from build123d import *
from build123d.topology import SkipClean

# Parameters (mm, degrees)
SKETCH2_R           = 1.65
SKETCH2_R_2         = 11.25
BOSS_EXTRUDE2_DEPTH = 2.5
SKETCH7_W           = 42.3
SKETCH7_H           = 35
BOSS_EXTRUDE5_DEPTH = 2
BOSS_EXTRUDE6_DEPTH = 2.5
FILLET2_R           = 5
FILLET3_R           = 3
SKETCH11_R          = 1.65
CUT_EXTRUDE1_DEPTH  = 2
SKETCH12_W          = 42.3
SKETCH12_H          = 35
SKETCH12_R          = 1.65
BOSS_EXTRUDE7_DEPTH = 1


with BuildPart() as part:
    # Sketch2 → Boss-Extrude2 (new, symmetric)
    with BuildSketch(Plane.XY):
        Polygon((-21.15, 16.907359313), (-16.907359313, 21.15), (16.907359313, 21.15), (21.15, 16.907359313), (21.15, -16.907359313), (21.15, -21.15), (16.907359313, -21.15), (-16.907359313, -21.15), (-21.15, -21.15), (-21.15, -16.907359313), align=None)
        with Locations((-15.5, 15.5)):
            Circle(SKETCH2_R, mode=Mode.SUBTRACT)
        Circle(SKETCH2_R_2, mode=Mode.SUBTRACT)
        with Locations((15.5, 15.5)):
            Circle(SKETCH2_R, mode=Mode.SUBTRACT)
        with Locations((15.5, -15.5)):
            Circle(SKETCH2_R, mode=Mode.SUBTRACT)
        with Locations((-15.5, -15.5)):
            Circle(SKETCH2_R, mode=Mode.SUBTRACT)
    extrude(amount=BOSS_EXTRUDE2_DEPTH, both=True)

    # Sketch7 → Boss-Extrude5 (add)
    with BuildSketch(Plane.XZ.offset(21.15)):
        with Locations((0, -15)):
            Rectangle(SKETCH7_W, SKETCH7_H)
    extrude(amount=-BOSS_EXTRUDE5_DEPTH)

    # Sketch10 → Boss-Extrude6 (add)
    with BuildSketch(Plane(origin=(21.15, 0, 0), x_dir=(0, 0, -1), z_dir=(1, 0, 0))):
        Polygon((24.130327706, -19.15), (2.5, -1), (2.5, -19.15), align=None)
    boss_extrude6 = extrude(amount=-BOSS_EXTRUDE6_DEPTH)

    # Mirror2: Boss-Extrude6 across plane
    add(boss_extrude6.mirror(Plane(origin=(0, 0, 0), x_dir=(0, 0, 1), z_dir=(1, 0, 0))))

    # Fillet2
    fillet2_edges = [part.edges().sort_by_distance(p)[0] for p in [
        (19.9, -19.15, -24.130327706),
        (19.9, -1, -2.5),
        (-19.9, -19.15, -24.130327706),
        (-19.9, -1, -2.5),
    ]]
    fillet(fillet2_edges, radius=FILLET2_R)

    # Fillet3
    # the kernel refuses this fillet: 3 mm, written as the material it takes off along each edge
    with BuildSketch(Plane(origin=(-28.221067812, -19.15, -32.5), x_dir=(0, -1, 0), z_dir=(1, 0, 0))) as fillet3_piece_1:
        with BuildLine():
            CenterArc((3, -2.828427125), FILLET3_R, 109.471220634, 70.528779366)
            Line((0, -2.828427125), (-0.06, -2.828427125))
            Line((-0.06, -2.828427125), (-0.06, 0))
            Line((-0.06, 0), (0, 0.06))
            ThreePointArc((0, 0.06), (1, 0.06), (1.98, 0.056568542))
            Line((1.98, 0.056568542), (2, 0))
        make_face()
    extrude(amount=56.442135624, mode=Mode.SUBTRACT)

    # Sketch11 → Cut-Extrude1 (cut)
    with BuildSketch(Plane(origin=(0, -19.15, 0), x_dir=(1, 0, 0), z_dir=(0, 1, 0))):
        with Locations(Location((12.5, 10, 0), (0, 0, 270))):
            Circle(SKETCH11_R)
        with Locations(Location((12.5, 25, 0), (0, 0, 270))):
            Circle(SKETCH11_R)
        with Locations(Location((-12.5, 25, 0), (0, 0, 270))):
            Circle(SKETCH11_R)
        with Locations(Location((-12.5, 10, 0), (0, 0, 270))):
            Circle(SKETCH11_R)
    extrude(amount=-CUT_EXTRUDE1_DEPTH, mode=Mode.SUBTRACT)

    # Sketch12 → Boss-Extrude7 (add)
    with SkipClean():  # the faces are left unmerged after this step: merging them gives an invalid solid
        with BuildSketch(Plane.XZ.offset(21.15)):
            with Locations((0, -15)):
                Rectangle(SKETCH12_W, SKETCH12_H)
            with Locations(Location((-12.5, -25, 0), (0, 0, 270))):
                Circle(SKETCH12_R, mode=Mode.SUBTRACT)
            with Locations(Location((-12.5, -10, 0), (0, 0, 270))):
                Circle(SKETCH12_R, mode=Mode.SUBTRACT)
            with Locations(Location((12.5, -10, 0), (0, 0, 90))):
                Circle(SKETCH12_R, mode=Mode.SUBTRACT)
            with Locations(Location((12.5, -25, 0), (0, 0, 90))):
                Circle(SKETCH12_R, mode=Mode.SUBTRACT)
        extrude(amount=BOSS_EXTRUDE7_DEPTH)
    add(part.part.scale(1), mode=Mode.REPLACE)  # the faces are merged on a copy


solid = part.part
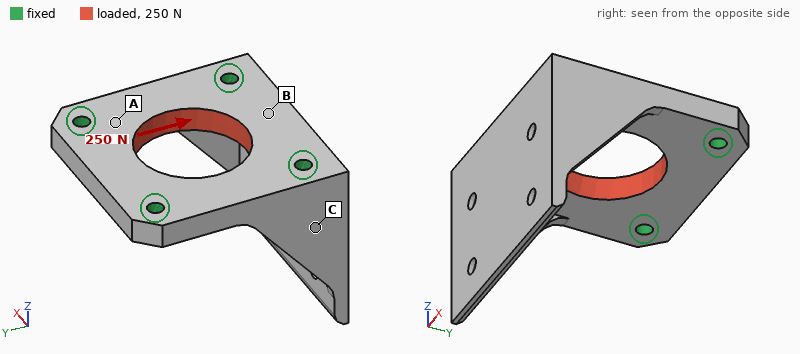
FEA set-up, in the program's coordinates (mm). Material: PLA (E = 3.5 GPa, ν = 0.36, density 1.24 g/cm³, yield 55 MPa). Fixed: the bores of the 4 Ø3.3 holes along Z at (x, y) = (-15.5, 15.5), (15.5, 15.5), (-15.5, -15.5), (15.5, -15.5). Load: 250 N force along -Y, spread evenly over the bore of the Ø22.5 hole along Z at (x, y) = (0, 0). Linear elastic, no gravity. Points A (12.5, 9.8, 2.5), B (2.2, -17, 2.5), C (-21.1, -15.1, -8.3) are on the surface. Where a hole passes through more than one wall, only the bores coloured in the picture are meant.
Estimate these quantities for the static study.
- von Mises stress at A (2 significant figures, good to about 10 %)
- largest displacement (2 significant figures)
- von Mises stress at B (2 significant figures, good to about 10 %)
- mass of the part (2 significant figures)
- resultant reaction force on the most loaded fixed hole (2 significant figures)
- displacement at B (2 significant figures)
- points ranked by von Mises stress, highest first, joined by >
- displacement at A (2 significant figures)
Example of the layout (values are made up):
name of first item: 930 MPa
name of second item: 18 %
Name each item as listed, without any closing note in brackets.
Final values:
von Mises stress at A: 1.1 MPa
largest displacement: 9.6 µm
von Mises stress at B: 0.55 MPa
mass of the part: 14 g
resultant reaction force on the most loaded fixed hole: 65 N
displacement at B: 6.9 µm
points ranked by von Mises stress, highest first, joined by >: A > B > C
displacement at A: 2.8 µm
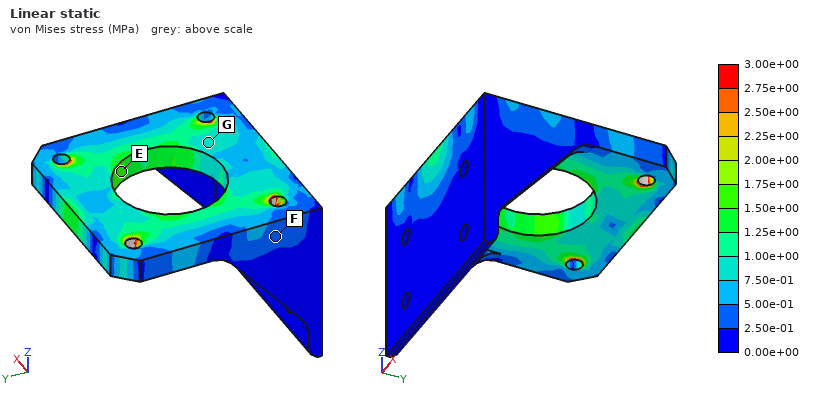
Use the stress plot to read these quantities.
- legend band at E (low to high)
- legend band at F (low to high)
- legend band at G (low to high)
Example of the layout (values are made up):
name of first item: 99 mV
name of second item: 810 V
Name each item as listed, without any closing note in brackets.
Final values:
legend band at E: 1.50e+00 to 1.75e+00 MPa
legend band at F: 2.50e-01 to 5.00e-01 MPa
legend band at G: 7.50e-01 to 1.00e+00 MPa
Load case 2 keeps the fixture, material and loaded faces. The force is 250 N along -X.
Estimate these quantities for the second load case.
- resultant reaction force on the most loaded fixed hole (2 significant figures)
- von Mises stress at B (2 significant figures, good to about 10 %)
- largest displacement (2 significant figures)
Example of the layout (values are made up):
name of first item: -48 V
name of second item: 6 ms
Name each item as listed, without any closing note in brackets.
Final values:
resultant reaction force on the most loaded fixed hole: 65 N
von Mises stress at B: 0.71 MPa
largest displacement: 9.1 µm
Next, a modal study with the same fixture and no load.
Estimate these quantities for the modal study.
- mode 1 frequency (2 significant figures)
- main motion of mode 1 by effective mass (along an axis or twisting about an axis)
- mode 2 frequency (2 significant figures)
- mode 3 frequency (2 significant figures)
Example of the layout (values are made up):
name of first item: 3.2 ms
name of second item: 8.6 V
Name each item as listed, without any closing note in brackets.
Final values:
mode 1 frequency: 1600 Hz
main motion of mode 1 by effective mass: along Y
mode 2 frequency: 3000 Hz
mode 3 frequency: 4900 Hz
